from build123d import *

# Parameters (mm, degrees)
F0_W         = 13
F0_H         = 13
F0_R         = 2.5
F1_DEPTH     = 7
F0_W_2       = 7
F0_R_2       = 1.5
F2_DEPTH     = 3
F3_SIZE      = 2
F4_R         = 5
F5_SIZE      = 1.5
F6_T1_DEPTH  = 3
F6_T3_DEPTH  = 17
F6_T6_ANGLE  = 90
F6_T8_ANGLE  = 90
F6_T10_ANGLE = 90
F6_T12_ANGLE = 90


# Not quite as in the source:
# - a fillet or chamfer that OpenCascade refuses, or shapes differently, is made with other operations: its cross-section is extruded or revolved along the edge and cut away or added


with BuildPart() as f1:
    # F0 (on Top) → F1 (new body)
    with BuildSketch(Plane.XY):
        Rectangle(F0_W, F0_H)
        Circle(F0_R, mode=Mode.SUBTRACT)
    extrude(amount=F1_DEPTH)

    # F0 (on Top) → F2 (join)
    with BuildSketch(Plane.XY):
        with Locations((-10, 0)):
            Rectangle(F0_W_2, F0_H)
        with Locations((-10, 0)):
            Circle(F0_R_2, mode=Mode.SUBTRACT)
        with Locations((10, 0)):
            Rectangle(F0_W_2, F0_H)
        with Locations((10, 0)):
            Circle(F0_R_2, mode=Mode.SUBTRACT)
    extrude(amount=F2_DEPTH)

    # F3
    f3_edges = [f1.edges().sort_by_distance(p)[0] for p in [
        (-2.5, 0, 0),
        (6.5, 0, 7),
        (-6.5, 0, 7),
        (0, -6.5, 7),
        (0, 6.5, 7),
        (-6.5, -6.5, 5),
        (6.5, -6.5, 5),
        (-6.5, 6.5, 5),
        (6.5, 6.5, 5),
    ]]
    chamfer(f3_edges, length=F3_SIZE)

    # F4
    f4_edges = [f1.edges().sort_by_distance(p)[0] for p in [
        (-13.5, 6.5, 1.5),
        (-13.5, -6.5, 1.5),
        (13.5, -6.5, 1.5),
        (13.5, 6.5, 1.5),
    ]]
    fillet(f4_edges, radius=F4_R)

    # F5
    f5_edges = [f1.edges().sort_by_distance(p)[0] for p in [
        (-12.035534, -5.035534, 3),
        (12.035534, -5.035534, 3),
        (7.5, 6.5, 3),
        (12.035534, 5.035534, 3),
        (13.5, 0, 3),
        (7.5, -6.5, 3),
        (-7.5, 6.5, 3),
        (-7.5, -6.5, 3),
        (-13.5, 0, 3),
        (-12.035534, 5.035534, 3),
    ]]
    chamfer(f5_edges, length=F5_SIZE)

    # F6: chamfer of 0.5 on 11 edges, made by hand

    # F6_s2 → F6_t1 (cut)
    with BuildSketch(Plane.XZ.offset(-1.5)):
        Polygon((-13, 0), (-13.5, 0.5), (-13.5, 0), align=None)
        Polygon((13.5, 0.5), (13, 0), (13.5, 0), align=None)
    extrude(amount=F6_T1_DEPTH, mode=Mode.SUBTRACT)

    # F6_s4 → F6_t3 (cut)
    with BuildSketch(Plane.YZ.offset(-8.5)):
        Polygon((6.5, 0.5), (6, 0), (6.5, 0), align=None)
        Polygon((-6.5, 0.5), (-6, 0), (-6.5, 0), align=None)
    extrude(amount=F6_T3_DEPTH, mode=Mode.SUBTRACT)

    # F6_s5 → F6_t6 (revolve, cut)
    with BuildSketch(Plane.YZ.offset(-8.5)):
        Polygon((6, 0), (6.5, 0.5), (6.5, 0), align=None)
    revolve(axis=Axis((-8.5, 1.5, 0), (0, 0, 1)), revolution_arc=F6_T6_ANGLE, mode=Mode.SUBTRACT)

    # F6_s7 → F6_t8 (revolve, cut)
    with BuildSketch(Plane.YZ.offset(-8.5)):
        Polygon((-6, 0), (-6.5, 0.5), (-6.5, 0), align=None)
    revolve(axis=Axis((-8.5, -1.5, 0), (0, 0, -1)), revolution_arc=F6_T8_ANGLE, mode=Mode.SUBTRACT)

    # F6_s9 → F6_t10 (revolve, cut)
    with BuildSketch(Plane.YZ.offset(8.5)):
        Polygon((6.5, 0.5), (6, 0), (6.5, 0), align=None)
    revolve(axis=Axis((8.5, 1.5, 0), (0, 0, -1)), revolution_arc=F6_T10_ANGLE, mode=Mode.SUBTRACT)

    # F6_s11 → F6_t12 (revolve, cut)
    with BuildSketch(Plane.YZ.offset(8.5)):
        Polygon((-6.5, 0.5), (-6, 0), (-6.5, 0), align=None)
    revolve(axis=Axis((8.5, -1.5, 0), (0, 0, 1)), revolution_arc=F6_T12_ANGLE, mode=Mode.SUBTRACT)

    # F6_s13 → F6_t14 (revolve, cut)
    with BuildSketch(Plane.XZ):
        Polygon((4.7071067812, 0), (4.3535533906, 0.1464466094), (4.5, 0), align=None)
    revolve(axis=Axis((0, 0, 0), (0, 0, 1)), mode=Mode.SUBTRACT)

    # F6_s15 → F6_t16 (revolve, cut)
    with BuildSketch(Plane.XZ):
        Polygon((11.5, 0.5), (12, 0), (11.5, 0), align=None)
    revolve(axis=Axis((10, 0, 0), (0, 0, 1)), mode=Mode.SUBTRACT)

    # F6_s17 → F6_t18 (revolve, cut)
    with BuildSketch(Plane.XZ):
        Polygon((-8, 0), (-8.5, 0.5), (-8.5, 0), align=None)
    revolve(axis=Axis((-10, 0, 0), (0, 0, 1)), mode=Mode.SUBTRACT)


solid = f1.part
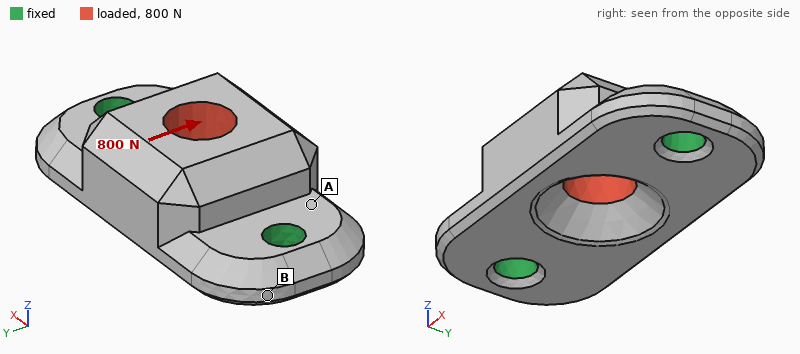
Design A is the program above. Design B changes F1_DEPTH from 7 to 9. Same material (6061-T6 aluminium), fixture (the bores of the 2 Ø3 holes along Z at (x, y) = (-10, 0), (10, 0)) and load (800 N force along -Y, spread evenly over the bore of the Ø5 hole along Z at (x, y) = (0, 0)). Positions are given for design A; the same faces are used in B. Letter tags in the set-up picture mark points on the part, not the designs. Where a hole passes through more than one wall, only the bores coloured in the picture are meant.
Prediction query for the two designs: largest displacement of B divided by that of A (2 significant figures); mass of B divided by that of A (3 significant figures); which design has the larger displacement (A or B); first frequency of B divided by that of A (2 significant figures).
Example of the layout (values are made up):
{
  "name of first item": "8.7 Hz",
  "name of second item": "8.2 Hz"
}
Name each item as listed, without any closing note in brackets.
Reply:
{
  "largest displacement of B divided by that of A": "1.5",
  "mass of B divided by that of A": "1.22",
  "which design has the larger displacement": "B",
  "first frequency of B divided by that of A": "0.77"
}
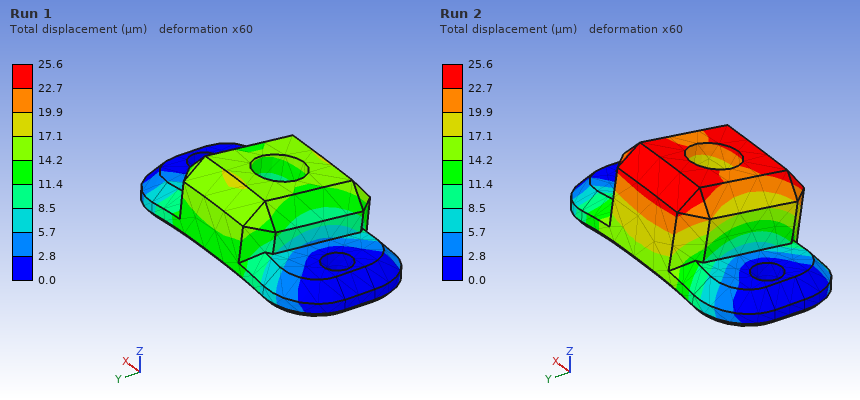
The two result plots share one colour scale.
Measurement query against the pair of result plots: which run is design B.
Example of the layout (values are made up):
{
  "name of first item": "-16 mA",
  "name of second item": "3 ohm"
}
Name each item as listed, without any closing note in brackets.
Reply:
{
  "which run is design B": "Run 2"
}
